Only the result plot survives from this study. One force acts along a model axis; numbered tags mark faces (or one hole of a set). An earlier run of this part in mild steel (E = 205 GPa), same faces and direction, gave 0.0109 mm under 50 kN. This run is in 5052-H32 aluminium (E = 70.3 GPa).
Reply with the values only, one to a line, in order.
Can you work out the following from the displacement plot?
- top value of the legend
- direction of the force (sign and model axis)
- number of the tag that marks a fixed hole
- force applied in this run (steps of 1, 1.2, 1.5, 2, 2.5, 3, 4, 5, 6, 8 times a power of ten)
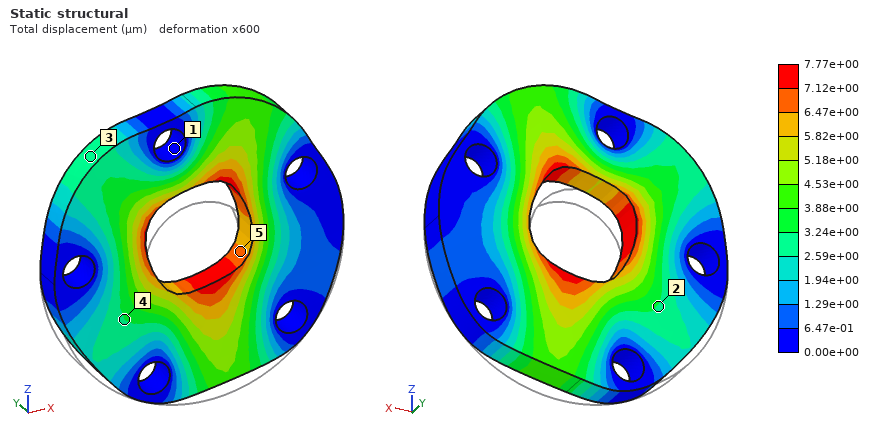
7.77e+00 µm
+Z
1
12 kN
